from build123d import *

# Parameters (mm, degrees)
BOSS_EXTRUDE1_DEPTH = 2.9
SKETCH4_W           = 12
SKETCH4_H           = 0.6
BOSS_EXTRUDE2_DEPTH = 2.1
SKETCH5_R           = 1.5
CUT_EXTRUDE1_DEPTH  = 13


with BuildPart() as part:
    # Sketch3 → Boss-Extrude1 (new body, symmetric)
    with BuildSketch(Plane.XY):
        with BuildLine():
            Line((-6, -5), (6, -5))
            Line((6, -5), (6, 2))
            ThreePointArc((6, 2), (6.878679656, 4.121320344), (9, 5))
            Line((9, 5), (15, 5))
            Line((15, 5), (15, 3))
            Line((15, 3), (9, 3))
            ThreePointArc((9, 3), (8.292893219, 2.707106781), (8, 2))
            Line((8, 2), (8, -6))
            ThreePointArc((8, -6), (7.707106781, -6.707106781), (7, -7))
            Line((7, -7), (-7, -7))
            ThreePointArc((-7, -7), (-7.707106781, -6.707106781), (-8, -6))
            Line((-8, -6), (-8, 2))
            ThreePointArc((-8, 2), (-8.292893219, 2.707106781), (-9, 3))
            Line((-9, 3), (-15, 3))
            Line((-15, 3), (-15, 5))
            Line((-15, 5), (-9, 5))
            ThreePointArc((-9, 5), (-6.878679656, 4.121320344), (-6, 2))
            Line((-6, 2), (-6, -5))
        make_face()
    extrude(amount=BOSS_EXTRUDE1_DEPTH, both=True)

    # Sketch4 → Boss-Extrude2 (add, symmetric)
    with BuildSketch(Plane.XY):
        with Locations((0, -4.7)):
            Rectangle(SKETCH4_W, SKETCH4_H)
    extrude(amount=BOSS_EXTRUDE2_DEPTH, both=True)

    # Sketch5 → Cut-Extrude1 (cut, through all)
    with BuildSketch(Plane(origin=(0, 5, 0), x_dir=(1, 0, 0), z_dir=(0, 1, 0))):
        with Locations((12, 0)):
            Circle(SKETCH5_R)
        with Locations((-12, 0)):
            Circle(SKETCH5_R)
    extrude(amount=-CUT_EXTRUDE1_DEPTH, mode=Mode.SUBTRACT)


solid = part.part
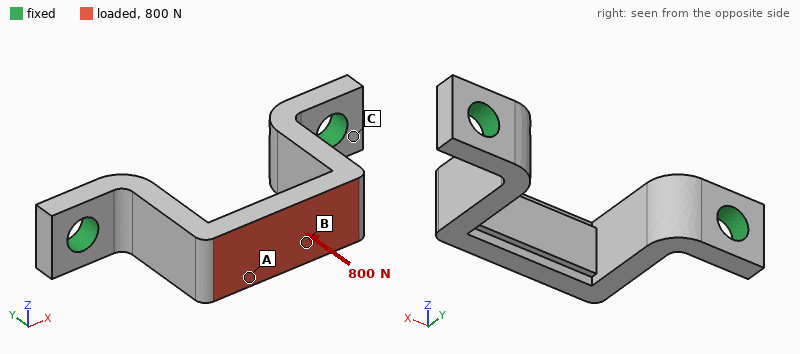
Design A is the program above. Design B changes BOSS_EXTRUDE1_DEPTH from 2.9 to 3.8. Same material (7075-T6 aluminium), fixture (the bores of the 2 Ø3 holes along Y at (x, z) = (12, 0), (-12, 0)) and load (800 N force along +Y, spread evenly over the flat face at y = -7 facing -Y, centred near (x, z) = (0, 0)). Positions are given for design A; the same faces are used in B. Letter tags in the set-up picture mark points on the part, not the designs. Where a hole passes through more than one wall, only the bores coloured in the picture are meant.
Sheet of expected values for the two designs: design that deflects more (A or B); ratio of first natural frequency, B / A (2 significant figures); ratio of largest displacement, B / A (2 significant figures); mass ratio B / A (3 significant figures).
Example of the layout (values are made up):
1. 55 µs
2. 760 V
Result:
1. A
2. 1.1
3. 0.85
4. 1.31
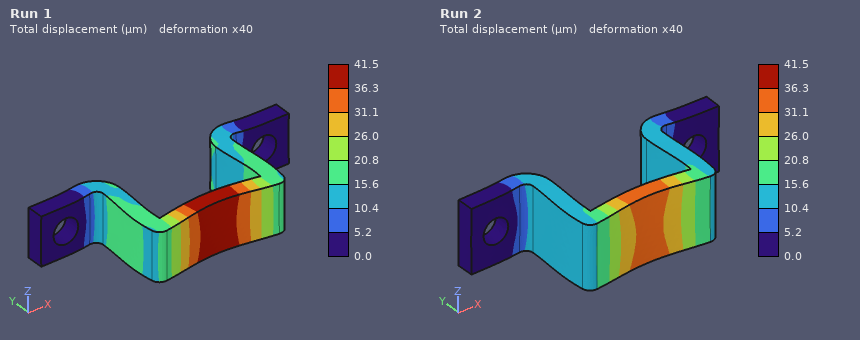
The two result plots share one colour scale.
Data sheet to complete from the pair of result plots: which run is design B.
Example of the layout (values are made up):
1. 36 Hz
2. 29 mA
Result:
1. Run 2
